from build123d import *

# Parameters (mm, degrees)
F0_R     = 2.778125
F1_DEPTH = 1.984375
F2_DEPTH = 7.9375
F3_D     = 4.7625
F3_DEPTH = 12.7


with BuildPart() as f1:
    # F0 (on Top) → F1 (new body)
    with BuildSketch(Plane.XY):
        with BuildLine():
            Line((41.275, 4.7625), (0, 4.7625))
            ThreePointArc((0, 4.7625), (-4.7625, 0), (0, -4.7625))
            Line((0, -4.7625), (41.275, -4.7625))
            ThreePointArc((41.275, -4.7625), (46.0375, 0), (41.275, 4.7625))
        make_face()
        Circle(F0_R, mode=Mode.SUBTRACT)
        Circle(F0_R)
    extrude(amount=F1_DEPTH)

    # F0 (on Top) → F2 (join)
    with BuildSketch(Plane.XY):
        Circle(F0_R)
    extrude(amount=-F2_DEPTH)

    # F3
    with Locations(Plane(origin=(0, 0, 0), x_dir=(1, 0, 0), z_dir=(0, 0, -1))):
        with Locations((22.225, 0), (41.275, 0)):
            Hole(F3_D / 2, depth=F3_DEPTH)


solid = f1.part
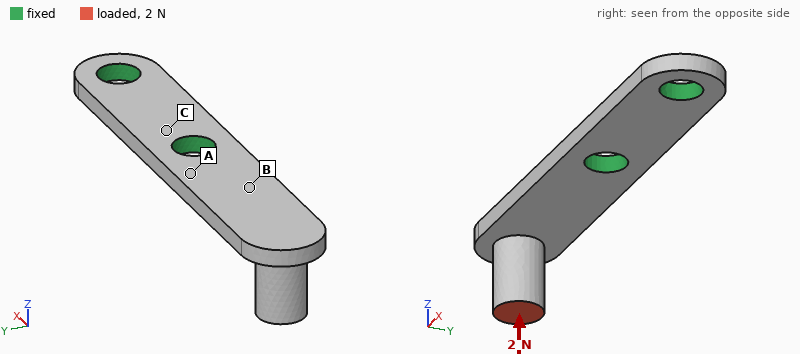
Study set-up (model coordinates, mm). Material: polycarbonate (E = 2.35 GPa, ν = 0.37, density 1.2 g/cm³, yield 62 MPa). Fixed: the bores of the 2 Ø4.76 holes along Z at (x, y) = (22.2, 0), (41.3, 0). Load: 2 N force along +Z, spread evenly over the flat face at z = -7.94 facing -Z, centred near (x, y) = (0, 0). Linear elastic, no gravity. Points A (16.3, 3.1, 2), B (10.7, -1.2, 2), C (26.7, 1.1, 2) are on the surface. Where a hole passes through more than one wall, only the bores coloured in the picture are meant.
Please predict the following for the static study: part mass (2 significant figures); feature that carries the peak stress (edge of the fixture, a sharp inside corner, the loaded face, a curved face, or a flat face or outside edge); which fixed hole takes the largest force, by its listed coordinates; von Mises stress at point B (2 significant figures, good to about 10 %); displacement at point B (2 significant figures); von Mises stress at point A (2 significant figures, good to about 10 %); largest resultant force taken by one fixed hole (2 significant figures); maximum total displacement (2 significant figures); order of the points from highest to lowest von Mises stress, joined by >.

1.3 g
a flat face or outside edge
(22.2, 0)
3.3 MPa
0.11 mm
5.0 MPa
2.0 N
0.52 mm
A > B > C
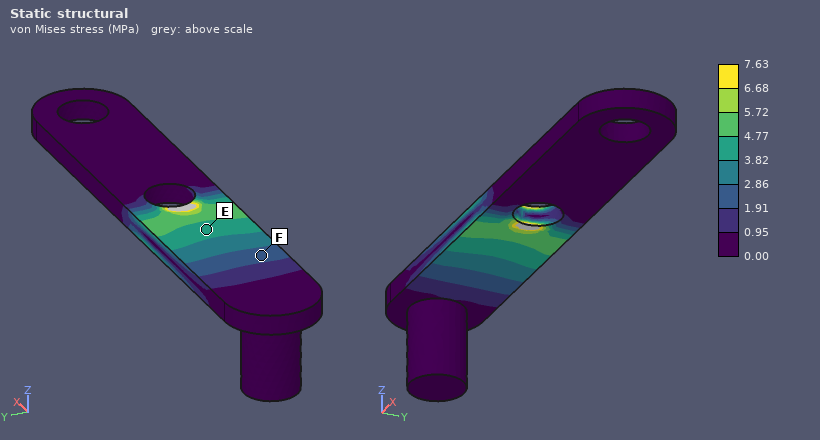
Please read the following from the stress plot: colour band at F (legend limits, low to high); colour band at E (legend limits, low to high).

1.91 to 2.86 MPa
3.82 to 4.77 MPa
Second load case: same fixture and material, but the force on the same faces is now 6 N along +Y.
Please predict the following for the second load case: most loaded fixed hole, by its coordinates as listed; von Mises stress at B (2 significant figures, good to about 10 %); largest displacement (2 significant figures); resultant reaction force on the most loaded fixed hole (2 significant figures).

(22.2, 0)
7.4 MPa
0.55 mm
7.3 N
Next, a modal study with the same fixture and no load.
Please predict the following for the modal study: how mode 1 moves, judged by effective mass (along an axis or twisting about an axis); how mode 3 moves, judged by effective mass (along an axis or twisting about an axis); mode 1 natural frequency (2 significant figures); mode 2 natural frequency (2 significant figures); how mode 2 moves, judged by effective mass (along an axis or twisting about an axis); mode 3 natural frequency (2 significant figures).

along Z
along Y
520 Hz
1500 Hz
along Y
2800 Hz
